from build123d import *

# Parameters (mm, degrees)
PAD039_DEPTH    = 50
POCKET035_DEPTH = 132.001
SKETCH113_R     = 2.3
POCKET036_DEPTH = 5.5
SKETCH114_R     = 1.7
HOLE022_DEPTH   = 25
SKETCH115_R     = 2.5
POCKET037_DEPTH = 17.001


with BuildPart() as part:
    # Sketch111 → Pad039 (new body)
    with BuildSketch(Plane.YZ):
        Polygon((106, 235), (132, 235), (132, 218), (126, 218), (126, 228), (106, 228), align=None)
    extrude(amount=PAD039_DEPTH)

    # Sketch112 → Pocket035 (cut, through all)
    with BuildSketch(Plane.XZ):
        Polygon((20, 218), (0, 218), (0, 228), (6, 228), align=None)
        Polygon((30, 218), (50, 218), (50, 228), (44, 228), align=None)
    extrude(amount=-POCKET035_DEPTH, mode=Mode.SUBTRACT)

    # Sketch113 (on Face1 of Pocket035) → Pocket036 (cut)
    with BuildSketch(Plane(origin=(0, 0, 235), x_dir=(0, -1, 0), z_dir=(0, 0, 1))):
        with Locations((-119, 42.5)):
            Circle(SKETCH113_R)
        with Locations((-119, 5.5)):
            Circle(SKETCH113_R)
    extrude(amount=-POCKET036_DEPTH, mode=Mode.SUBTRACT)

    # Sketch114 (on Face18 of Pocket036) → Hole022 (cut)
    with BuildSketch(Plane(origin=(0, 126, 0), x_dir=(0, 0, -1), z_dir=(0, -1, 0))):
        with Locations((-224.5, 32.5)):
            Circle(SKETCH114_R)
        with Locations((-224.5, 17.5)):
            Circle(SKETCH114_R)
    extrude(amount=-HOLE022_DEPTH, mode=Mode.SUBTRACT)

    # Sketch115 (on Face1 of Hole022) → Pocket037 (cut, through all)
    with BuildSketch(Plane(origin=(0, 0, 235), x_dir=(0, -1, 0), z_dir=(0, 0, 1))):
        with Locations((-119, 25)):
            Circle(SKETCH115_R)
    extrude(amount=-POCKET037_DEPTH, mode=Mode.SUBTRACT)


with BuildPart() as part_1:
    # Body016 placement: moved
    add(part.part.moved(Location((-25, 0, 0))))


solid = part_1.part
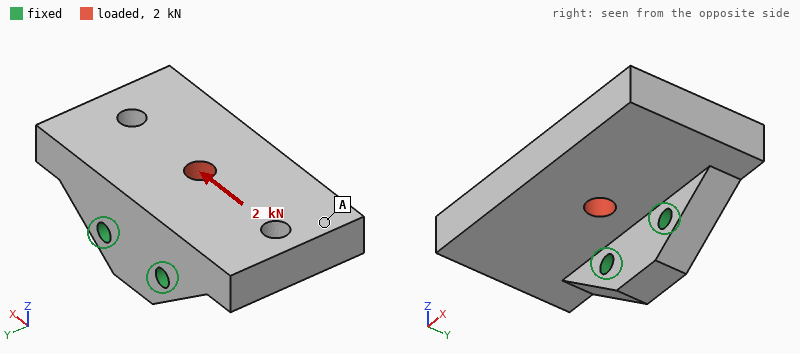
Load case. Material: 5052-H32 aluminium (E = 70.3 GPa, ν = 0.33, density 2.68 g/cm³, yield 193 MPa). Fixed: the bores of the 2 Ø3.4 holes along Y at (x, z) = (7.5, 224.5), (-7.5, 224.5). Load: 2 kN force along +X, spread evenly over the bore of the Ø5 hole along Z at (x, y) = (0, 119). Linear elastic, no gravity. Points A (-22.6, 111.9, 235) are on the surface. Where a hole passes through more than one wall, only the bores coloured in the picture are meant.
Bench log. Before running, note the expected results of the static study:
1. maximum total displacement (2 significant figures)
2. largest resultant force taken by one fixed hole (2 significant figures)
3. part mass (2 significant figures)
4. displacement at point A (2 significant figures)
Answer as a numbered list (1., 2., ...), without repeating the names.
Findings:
1. 31 µm
2. 1.6 kN
3. 27 g
4. 26 µm
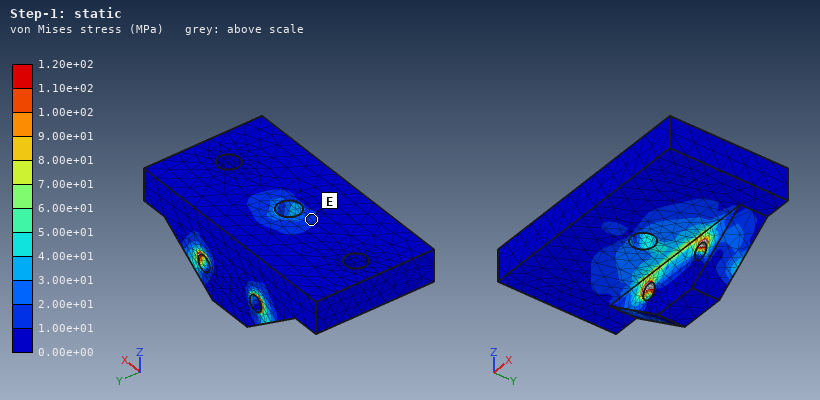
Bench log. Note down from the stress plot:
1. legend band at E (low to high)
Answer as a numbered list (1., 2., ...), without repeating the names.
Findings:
1. 1.00e+01 to 2.00e+01 MPa
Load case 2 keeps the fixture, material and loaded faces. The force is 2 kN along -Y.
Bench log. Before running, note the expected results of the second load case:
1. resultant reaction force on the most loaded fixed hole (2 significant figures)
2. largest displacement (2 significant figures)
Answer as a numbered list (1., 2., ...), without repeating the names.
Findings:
1. 1.0 kN
2. 42 µm
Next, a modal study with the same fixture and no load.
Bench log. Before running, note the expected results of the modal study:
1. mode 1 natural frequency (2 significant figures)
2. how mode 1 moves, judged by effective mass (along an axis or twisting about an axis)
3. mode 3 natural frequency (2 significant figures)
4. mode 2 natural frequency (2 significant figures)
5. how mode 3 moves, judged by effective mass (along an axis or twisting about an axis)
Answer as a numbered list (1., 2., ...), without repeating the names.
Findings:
1. 5200 Hz
2. along Z
3. 9800 Hz
4. 7500 Hz
5. along X
